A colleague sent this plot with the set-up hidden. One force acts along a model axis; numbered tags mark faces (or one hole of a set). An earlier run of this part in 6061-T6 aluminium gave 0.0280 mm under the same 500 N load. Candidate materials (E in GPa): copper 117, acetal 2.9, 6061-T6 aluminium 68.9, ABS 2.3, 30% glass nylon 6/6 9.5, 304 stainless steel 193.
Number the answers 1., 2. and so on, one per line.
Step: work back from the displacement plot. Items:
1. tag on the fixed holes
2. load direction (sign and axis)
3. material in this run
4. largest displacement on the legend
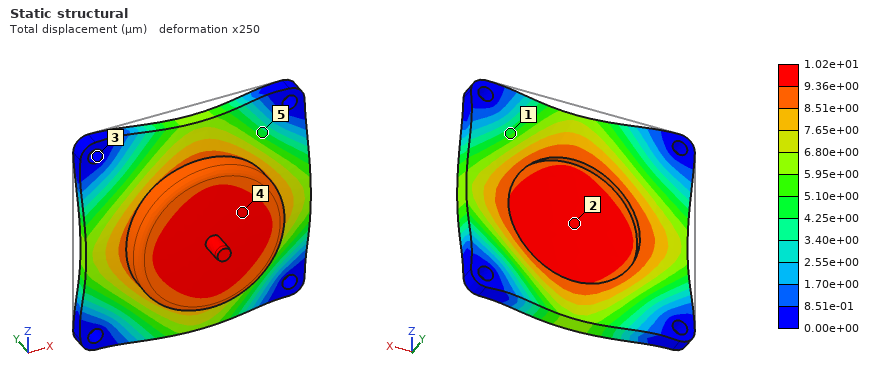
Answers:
1. 3
2. -Y
3. 304 stainless steel
4. 1.02e+01 µm
